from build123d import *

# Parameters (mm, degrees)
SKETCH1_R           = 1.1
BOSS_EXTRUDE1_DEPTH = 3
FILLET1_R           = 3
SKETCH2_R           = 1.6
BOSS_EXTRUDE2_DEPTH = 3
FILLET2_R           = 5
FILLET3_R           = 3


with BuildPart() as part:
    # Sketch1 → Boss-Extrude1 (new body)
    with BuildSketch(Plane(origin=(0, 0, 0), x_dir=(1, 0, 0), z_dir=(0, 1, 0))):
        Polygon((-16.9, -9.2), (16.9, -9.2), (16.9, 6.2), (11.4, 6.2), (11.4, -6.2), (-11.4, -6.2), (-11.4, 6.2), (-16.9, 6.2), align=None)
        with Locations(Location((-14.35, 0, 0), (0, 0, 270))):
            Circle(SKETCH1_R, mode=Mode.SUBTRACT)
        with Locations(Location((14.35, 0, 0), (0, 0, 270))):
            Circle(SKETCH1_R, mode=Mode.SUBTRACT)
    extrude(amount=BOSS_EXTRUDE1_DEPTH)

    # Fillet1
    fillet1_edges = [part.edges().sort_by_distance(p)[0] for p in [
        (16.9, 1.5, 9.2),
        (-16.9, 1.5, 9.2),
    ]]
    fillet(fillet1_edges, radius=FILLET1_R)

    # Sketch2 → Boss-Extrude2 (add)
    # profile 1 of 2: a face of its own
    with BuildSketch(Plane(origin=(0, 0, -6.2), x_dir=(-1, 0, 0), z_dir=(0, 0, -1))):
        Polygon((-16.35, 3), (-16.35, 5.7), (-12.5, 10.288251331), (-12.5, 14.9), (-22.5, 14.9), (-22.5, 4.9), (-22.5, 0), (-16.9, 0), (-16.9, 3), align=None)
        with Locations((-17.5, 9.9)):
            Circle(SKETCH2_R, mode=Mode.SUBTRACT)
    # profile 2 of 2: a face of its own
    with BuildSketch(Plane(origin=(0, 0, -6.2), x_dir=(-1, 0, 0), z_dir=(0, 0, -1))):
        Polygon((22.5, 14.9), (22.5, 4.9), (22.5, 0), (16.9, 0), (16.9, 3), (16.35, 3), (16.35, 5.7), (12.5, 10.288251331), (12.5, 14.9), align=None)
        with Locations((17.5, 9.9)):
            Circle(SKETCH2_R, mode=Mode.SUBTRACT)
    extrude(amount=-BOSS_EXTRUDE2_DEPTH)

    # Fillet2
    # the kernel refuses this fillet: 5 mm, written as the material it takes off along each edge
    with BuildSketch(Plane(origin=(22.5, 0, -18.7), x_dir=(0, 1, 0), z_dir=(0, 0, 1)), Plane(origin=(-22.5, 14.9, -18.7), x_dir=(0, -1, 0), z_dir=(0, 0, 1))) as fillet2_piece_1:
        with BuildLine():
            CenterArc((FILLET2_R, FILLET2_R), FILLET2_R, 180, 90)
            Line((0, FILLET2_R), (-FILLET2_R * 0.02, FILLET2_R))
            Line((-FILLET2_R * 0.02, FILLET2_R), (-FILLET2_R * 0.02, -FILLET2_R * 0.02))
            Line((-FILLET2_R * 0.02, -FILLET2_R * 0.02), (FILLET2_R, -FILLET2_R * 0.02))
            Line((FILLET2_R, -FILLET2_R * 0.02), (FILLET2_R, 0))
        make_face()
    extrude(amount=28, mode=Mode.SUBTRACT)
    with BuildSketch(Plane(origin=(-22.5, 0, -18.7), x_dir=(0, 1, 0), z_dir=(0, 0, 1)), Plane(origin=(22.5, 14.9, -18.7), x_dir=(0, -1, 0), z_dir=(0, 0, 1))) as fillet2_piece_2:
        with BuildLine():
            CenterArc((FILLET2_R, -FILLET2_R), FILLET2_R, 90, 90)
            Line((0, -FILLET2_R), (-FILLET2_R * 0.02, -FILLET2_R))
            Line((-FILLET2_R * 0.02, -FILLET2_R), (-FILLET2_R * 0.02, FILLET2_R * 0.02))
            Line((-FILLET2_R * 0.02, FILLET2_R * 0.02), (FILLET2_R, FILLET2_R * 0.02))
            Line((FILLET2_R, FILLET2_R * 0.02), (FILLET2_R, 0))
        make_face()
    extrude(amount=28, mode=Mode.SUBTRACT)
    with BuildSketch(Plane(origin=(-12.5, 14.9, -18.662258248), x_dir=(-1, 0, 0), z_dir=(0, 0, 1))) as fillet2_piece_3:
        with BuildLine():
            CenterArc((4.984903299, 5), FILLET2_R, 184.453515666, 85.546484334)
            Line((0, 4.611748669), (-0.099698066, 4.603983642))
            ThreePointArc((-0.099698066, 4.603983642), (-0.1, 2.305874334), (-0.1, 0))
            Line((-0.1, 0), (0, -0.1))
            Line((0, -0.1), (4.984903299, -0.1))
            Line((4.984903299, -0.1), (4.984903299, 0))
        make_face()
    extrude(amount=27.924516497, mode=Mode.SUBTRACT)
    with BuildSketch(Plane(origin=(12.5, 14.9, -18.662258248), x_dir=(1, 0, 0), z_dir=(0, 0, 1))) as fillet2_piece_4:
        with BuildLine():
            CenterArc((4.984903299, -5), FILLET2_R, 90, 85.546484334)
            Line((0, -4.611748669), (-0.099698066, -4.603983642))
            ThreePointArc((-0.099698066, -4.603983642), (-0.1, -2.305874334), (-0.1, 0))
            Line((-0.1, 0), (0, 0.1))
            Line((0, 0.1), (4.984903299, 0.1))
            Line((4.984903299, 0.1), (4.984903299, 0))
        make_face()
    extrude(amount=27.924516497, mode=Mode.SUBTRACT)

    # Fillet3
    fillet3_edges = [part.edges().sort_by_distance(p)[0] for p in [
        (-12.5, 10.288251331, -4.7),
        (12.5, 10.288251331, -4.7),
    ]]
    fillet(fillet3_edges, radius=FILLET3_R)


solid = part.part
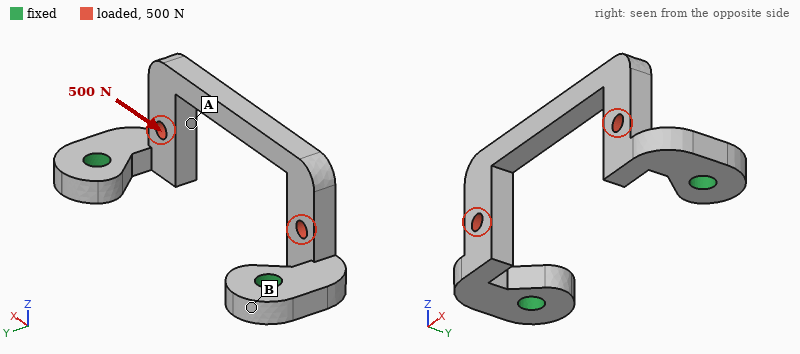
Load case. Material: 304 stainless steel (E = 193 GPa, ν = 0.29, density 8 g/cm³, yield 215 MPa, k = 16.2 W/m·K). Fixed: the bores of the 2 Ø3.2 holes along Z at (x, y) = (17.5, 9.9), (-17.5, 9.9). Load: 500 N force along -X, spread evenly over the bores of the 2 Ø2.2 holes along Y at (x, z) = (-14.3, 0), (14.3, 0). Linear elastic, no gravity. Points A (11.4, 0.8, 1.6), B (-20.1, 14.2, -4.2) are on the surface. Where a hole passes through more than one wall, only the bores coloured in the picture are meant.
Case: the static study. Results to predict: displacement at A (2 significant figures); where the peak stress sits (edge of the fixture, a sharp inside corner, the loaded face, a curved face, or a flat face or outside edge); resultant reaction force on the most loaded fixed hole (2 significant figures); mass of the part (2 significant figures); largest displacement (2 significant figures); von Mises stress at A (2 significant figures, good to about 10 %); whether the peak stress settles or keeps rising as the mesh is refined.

21 µm
a sharp inside corner
250 N
9.8 g
29 µm
56 MPa
keeps rising
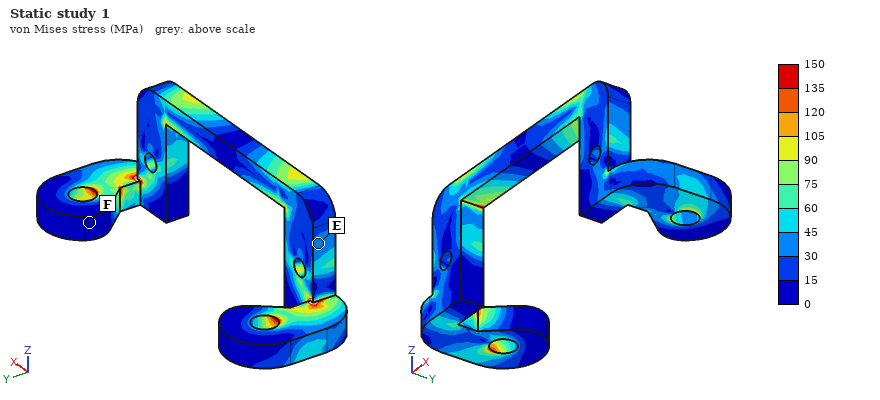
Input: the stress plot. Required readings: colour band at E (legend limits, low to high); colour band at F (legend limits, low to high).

30 to 45 MPa
0 to 15 MPa
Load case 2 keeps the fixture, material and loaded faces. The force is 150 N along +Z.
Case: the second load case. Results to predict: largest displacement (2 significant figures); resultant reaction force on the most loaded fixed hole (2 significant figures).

14 µm
77 N
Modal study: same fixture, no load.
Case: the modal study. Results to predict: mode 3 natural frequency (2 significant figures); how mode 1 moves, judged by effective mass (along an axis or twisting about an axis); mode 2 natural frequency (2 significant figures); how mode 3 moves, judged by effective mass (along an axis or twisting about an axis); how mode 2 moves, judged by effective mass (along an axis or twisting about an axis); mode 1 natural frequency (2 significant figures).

7700 Hz
along Y
7400 Hz
along X
along X
3800 Hz
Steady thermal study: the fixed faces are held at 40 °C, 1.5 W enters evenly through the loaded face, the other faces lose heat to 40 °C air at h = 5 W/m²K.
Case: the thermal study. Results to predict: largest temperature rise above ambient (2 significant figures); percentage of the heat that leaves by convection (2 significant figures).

40 K
10 %
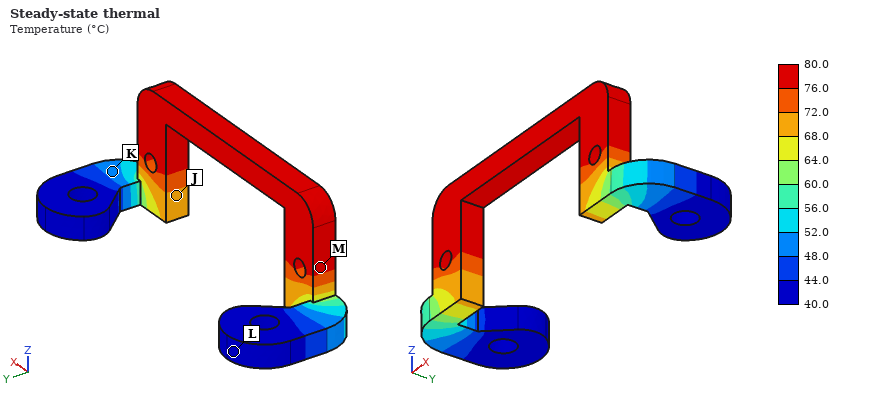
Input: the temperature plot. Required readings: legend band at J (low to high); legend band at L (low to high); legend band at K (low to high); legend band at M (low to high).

68.0 to 72.0 °C
40.0 to 44.0 °C
48.0 to 52.0 °C
76.0 to 80.0 °C
